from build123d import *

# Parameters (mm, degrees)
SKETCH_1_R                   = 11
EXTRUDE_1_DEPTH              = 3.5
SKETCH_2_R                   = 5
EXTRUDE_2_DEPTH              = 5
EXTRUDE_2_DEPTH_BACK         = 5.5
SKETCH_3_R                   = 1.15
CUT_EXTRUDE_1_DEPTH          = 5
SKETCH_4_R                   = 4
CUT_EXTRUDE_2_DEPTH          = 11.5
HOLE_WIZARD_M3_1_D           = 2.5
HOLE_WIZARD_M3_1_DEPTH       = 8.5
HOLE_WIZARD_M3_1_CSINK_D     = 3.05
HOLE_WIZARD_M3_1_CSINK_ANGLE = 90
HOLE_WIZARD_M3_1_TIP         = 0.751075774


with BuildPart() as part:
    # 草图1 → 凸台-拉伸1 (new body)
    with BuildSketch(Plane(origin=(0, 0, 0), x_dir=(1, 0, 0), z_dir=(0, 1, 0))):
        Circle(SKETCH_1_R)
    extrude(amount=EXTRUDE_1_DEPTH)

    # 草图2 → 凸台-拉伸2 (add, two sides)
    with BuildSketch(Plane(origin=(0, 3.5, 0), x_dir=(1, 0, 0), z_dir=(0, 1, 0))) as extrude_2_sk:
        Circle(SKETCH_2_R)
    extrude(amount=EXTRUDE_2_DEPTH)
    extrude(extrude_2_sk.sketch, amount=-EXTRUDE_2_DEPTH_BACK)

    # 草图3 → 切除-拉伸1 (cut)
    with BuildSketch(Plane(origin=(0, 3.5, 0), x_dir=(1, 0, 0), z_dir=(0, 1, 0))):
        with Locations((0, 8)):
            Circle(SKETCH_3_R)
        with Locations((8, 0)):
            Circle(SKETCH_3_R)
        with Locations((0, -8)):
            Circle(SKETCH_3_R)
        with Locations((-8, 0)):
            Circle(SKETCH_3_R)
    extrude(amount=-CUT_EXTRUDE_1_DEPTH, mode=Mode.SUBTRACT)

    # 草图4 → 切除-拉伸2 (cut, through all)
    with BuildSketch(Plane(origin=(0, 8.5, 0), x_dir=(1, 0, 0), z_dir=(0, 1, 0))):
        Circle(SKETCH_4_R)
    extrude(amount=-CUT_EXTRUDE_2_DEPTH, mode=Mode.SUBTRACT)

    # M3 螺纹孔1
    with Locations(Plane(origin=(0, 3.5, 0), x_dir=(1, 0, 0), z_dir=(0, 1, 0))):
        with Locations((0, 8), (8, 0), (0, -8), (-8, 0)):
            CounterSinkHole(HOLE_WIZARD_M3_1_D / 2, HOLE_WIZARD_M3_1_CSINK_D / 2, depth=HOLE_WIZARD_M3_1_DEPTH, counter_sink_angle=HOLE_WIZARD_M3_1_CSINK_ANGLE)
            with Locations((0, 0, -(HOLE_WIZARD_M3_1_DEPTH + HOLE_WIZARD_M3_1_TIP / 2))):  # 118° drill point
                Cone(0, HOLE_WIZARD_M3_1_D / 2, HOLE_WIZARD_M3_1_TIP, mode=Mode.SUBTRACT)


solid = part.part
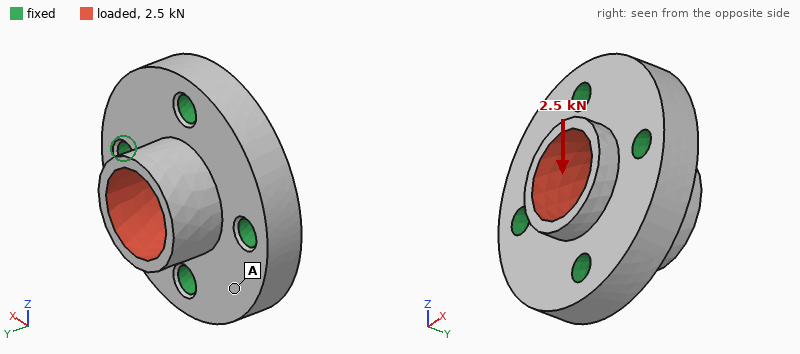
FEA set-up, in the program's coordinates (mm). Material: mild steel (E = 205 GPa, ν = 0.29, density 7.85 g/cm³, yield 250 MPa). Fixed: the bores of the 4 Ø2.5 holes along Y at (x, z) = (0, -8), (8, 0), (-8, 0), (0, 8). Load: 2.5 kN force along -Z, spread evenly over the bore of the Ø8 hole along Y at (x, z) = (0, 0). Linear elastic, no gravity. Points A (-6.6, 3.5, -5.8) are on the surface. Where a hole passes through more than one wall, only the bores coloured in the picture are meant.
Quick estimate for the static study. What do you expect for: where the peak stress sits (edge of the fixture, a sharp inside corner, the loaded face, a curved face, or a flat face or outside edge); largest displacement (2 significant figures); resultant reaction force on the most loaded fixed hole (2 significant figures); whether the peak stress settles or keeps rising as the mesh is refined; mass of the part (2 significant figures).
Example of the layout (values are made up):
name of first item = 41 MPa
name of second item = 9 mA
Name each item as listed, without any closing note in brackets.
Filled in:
where the peak stress sits = edge of the fixture
largest displacement = 5.7 µm
resultant reaction force on the most loaded fixed hole = 740 N
whether the peak stress settles or keeps rising as the mesh is refined = keeps rising
mass of the part = 10 g
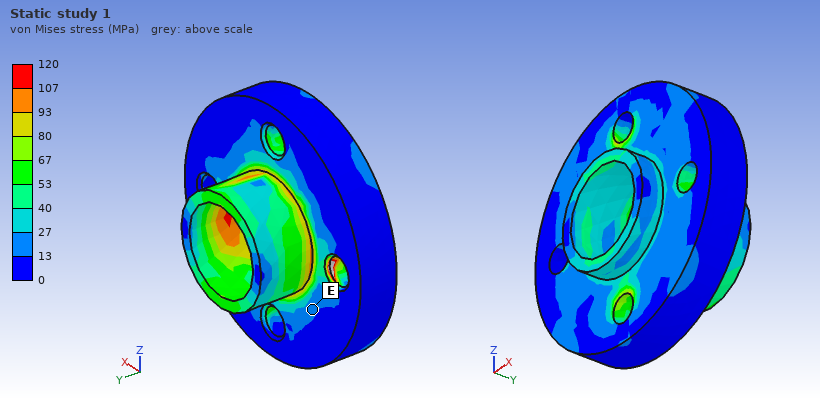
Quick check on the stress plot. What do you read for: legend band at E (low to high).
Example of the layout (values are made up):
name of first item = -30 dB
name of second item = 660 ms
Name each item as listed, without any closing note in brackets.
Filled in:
legend band at E = 13 to 27 MPa
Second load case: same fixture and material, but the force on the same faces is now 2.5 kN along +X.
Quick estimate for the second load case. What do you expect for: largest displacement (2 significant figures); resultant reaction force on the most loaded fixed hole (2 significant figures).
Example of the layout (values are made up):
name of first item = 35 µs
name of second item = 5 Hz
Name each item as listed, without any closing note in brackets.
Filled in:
largest displacement = 5.7 µm
resultant reaction force on the most loaded fixed hole = 740 N
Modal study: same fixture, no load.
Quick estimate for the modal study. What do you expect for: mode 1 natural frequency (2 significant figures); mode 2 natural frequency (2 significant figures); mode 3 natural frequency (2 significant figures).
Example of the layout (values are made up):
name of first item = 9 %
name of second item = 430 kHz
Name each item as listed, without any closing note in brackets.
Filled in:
mode 1 natural frequency = 65 kHz
mode 2 natural frequency = 72 kHz
mode 3 natural frequency = 75 kHz
